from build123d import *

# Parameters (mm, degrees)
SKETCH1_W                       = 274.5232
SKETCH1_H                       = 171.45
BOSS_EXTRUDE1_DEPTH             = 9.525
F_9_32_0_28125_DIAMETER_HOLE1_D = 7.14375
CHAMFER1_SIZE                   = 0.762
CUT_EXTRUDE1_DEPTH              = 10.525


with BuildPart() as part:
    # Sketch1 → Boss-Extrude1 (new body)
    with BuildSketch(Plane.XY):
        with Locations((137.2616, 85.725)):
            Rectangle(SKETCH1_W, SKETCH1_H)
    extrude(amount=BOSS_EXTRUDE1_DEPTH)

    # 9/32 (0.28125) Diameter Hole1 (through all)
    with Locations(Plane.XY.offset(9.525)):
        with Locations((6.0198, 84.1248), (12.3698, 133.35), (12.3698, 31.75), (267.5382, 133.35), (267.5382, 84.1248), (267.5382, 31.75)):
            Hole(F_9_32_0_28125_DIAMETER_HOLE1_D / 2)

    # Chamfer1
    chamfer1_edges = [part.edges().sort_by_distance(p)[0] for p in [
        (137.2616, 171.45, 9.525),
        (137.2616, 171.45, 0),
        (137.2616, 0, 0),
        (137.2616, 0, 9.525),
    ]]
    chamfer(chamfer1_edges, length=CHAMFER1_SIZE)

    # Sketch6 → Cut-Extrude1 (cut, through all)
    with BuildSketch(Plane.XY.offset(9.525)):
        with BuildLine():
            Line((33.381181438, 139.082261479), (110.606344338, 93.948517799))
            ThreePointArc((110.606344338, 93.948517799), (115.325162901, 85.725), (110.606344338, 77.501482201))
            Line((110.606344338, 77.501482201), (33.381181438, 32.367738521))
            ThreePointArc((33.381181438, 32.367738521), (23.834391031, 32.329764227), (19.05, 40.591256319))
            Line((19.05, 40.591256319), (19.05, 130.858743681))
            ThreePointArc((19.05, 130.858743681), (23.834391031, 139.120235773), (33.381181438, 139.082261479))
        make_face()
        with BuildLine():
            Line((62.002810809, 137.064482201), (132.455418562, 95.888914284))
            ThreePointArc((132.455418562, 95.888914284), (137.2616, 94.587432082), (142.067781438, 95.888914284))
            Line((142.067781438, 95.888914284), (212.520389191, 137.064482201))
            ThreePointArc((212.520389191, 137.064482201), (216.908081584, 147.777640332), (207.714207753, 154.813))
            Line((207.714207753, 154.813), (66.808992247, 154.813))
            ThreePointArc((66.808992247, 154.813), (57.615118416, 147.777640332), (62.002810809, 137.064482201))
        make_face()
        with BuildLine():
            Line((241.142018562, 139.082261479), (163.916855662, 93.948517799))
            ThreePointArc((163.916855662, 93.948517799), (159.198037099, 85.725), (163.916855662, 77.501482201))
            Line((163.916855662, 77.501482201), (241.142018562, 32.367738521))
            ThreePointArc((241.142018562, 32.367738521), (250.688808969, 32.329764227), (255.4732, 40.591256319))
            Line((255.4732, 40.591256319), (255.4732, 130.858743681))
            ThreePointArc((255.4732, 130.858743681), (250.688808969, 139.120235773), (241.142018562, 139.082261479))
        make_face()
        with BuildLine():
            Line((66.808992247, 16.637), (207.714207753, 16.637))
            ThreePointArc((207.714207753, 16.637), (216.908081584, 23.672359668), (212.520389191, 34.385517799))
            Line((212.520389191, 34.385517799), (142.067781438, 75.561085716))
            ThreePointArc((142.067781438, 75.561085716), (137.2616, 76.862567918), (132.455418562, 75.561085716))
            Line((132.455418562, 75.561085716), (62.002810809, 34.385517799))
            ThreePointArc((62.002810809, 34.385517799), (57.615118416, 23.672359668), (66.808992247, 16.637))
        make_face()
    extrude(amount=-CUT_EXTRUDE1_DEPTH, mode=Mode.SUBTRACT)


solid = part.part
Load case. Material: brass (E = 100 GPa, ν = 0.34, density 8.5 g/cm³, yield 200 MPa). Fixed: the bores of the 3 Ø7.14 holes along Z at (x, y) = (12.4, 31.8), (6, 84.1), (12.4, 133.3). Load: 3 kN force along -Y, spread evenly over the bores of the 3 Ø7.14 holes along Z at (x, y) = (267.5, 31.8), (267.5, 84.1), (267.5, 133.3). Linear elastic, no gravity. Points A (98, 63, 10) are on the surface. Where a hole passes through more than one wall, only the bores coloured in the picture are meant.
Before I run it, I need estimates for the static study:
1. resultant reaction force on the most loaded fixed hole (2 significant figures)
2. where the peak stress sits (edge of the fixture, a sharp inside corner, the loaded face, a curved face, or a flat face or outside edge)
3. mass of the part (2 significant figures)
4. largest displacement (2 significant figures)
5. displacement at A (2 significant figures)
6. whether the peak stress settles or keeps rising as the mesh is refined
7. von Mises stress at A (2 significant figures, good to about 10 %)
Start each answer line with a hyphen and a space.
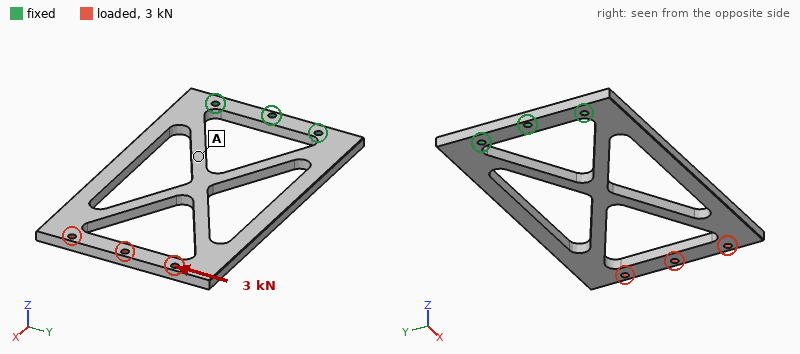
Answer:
- 6.5 kN
- edge of the fixture
- 1.8 kg
- 0.40 mm
- 0.13 mm
- keeps rising
- 28 MPa
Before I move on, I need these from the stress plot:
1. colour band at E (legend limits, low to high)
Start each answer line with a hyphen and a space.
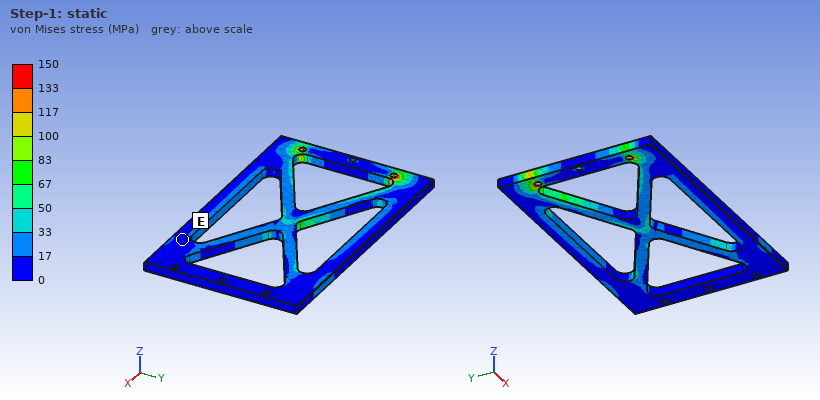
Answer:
- 0 to 17 MPa
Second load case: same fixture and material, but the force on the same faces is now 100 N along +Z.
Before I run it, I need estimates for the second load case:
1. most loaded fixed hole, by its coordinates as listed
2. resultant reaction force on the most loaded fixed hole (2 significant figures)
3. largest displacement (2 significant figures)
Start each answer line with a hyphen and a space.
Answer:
- (12.4, 31.8)
- 57 N
- 1.5 mm
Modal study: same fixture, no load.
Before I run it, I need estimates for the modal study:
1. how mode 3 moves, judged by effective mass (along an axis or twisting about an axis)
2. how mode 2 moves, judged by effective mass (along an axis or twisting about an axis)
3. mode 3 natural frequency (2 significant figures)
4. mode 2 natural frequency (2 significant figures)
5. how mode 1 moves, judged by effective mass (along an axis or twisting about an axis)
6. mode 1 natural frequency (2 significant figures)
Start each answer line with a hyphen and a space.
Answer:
- along Z
- twisting about X
- 390 Hz
- 170 Hz
- along Z
- 58 Hz
